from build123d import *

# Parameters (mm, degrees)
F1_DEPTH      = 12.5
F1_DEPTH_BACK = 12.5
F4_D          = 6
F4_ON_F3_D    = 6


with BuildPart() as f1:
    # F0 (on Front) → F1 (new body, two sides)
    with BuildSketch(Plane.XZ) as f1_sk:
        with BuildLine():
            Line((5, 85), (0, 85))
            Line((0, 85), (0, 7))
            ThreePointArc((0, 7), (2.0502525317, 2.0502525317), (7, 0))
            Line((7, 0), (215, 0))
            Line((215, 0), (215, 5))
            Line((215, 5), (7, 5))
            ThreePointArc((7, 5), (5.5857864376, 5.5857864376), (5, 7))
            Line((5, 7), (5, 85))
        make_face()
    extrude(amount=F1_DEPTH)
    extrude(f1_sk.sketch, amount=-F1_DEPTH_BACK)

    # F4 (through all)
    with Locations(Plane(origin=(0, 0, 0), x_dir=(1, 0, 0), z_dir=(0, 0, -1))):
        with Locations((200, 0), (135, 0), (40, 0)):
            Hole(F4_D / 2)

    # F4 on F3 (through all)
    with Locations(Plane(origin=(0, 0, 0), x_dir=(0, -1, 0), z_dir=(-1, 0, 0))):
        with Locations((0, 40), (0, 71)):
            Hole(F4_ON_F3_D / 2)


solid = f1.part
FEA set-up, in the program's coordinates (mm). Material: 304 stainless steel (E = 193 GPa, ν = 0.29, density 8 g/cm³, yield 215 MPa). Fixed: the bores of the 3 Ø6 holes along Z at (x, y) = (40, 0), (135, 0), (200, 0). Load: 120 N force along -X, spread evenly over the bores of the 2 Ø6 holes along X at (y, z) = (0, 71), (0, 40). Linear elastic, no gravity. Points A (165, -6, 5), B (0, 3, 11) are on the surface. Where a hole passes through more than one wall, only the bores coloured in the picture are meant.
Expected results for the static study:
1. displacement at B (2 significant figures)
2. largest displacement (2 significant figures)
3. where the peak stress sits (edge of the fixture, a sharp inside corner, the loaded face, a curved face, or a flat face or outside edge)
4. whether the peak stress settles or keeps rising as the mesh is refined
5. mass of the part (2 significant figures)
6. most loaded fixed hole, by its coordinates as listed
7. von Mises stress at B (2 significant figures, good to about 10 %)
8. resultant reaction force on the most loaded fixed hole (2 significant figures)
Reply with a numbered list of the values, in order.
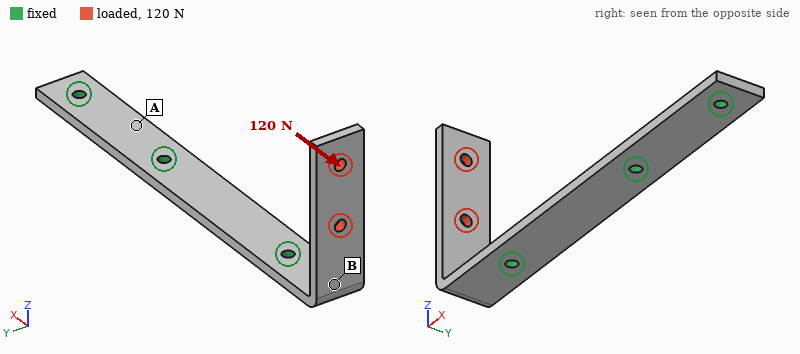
1. 0.11 mm
2. 0.59 mm
3. edge of the fixture
4. keeps rising
5. 290 g
6. (40, 0)
7. 46 MPa
8. 110 N
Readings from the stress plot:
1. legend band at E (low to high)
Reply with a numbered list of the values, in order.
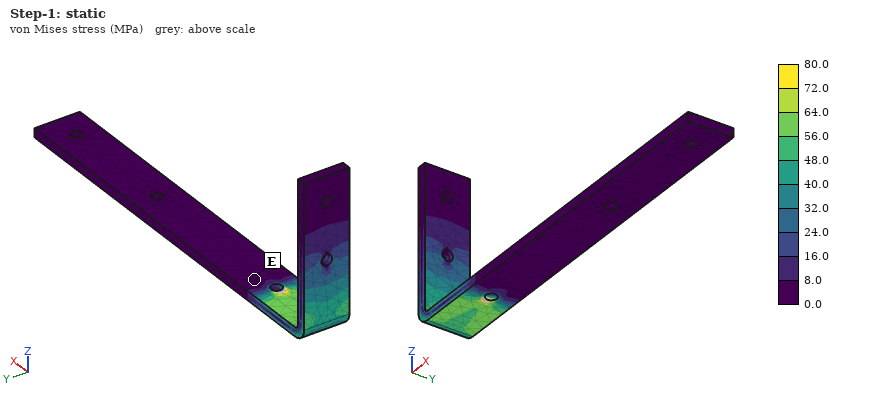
1. 0.0 to 8.0 MPa
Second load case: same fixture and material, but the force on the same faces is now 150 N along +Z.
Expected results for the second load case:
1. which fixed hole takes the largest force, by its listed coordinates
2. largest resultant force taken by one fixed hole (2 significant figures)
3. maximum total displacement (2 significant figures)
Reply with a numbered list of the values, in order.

1. (40, 0)
2. 150 N
3. 0.17 mm
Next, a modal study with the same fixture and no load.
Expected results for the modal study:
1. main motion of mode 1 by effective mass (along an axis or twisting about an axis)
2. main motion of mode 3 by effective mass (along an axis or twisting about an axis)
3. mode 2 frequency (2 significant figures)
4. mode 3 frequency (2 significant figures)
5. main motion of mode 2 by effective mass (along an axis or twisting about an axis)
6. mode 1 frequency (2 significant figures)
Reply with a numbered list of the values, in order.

1. along X
2. along Z
3. 520 Hz
4. 1300 Hz
5. along Y
6. 350 Hz
